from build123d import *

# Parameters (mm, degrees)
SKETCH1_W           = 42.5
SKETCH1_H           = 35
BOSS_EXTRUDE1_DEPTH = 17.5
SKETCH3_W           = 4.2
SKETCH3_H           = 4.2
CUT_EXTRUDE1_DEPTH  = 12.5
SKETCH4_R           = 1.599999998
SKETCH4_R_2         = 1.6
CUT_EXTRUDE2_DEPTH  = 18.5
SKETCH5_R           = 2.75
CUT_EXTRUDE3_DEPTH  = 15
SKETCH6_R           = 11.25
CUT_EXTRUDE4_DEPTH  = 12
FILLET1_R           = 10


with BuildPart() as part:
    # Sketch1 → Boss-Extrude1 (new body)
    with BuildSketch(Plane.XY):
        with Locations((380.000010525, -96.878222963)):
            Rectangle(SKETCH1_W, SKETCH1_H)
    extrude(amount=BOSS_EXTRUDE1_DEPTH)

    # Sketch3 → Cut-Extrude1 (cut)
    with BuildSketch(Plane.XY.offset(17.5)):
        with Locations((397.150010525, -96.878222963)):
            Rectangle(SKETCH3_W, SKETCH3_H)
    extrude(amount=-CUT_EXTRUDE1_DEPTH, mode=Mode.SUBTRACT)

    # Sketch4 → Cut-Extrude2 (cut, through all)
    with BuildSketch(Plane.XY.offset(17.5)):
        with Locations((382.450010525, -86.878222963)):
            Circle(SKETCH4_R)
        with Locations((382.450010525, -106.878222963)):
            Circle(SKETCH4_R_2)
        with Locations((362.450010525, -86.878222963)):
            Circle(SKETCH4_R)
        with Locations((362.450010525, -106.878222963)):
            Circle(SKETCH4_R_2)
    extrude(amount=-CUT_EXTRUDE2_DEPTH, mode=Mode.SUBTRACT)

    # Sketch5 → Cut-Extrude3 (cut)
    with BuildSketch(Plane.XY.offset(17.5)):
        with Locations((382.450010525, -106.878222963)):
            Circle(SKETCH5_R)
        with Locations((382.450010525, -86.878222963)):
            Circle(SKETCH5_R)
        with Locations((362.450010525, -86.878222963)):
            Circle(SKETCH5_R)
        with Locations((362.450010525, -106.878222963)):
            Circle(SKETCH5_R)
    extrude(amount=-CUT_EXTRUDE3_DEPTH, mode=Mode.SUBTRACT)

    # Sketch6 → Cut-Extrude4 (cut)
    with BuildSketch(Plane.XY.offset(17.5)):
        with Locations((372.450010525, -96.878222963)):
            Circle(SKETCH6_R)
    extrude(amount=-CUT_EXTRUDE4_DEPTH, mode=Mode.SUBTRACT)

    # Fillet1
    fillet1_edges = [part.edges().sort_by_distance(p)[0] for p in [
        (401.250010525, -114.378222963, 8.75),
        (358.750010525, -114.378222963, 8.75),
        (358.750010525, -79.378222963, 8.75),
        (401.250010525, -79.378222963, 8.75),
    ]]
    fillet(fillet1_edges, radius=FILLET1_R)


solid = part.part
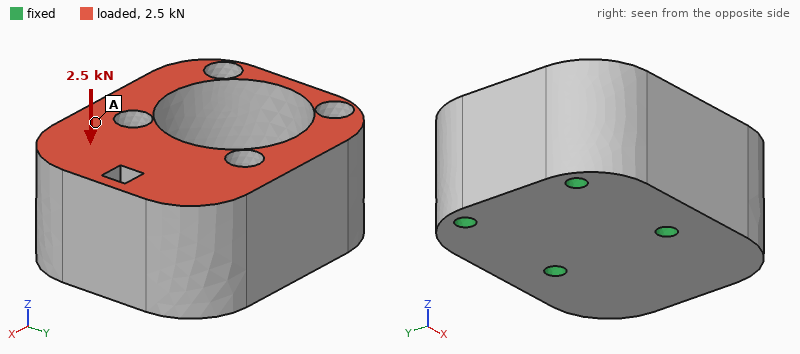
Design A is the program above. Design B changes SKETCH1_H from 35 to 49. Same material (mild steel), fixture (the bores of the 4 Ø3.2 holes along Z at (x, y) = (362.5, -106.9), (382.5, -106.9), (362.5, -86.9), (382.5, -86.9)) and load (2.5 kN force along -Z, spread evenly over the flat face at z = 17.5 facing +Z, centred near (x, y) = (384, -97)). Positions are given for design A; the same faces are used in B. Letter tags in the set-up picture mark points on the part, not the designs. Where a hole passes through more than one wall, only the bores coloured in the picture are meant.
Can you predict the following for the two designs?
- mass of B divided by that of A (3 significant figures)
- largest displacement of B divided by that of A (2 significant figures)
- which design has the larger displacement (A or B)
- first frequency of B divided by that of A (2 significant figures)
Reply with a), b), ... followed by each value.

a) 1.58
b) 0.72
c) A
d) 0.87
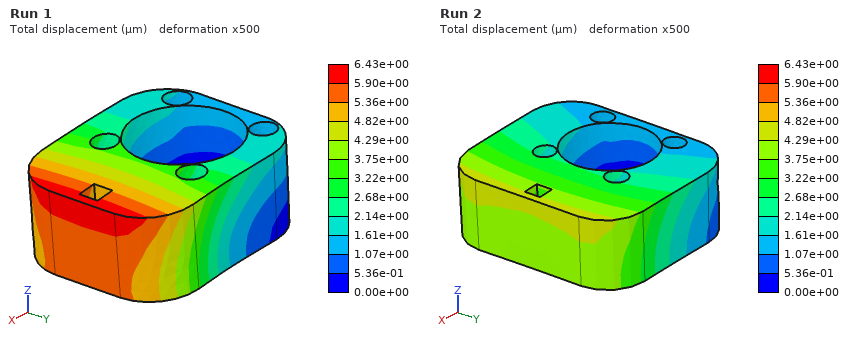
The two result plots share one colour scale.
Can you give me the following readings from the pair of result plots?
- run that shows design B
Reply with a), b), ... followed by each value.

a) Run 2
